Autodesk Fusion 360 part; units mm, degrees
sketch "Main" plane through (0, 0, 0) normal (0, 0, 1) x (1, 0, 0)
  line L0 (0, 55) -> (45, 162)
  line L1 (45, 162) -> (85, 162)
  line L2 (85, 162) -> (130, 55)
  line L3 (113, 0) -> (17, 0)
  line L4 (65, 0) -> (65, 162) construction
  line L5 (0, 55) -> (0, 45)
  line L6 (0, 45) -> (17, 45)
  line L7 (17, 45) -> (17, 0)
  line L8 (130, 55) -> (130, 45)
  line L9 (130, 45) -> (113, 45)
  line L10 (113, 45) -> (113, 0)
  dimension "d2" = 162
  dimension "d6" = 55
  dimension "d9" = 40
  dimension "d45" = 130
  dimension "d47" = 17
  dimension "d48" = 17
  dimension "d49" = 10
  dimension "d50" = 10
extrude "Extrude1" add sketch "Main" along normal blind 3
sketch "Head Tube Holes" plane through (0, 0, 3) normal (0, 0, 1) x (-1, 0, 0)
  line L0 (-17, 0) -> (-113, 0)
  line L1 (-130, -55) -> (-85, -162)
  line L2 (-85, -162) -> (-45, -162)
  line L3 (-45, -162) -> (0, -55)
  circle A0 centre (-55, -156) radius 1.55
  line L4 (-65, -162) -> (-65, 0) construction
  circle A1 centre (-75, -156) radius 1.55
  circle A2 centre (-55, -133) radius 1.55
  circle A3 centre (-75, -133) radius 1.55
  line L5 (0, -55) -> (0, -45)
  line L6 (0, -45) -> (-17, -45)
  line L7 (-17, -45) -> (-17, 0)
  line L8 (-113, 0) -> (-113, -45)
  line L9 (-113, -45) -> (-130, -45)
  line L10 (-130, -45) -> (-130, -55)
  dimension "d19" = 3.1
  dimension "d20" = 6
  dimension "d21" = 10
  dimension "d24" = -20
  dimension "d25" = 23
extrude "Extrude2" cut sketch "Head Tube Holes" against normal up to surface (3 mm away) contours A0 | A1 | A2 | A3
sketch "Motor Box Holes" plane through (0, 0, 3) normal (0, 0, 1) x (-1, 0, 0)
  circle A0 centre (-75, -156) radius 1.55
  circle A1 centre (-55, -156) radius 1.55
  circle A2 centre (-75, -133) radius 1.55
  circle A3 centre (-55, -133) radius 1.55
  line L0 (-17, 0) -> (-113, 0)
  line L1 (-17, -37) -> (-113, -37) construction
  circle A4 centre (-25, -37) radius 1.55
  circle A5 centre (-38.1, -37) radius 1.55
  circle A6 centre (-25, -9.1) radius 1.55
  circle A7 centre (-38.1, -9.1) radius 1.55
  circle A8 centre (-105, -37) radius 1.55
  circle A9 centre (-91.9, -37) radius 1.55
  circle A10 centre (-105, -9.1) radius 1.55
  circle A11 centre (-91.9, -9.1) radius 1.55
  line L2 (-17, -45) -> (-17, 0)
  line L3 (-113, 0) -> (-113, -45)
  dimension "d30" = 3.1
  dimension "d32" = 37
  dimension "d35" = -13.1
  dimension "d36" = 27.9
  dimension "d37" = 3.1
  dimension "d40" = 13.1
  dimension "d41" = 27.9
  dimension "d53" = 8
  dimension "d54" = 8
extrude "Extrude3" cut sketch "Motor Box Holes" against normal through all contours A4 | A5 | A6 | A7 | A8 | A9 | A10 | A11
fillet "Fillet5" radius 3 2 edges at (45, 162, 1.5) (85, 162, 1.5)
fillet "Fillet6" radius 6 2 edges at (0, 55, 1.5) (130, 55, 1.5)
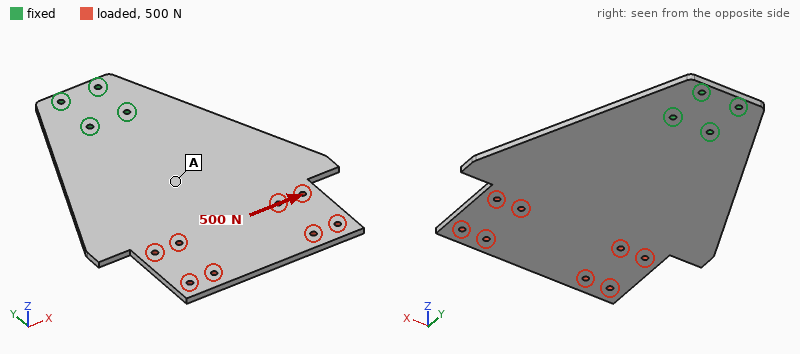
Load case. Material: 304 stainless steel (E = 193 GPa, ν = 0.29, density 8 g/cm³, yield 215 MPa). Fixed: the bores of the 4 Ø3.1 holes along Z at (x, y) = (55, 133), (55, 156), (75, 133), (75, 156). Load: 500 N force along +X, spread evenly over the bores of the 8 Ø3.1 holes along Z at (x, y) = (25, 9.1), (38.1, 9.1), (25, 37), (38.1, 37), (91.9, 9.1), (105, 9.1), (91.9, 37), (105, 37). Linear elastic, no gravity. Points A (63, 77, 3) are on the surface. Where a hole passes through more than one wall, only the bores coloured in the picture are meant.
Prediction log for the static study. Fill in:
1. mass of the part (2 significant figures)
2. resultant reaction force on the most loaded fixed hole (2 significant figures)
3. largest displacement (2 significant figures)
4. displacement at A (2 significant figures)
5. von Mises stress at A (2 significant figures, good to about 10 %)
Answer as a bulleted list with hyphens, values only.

- 350 g
- 1.3 kN
- 38 µm
- 14 µm
- 5.8 MPa
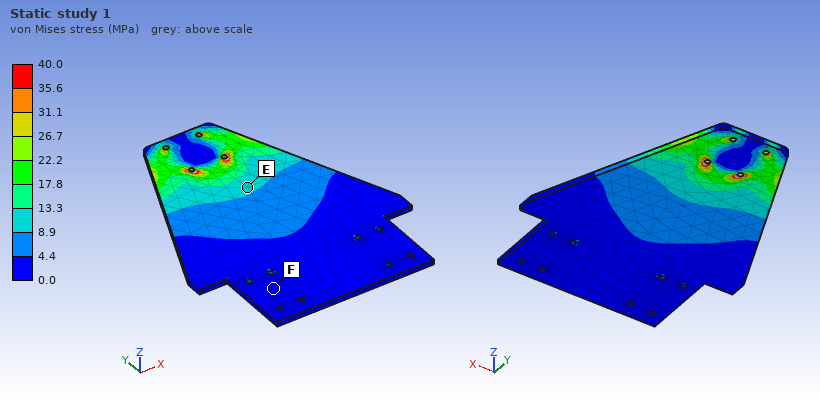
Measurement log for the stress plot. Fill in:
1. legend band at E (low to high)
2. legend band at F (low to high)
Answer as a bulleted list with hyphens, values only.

- 8.9 to 13.3 MPa
- 0.0 to 4.4 MPa
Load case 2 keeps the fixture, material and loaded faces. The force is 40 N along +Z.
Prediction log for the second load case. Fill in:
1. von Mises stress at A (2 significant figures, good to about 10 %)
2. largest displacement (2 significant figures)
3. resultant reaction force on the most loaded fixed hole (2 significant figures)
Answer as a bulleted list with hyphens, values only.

- 12 MPa
- 0.67 mm
- 61 N
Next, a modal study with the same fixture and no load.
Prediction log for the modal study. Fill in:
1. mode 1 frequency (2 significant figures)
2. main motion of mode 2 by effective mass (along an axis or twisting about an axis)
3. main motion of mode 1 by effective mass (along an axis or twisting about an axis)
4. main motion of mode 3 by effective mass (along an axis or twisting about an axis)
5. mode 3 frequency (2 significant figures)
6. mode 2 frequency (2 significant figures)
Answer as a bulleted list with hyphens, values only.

- 120 Hz
- twisting about Y
- along Z
- along Z
- 710 Hz
- 310 Hz
